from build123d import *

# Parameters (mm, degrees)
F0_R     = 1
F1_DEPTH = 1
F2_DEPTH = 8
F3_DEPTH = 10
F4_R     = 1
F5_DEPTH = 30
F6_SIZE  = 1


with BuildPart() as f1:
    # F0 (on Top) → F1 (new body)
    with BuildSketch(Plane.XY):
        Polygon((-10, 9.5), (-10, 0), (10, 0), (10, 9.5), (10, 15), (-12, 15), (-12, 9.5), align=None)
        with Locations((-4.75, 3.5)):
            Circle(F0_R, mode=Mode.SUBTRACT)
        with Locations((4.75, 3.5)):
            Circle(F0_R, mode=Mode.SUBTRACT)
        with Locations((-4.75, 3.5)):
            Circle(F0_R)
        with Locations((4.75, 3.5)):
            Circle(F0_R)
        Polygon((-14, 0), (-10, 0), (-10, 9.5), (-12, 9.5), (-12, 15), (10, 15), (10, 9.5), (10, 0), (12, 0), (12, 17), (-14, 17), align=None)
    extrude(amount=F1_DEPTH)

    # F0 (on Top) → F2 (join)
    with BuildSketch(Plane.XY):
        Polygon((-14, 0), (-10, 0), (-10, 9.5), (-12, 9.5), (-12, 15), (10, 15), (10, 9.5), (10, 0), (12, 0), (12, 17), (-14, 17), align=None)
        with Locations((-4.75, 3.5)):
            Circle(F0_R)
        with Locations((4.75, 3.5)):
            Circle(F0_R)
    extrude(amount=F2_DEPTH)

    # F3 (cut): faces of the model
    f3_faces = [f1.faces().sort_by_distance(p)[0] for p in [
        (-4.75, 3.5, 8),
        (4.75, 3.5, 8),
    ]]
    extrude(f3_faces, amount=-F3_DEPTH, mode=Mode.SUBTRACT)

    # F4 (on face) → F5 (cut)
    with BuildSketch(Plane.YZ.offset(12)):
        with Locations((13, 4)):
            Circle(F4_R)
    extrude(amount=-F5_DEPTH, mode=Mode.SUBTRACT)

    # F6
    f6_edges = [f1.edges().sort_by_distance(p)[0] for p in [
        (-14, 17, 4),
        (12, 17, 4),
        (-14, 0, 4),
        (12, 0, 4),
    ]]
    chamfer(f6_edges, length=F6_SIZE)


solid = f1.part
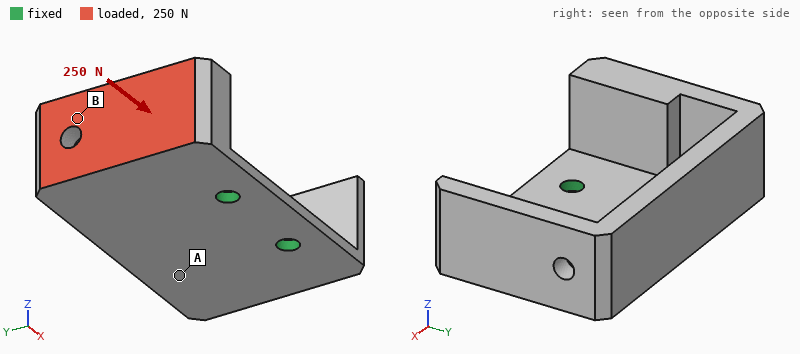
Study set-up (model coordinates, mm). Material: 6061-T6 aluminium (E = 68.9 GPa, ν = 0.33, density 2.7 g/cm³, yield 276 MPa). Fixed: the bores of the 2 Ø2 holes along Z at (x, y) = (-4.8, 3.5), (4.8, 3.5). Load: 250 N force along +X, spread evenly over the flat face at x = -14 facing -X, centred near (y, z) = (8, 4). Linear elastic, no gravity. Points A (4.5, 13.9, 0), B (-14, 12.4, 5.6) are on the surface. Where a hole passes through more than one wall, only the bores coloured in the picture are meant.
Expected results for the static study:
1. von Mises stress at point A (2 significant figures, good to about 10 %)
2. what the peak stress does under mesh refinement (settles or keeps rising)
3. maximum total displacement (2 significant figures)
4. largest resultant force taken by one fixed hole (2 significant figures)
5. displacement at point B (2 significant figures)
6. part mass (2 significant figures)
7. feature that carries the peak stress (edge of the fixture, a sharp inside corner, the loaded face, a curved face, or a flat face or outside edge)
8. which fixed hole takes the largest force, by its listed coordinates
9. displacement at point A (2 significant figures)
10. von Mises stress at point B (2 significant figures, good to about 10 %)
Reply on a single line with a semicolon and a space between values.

24 MPa; keeps rising; 0.20 mm; 220 N; 0.18 mm; 3.6 g; edge of the fixture; (-4.8, 3.5); 0.044 mm; 60 MPa
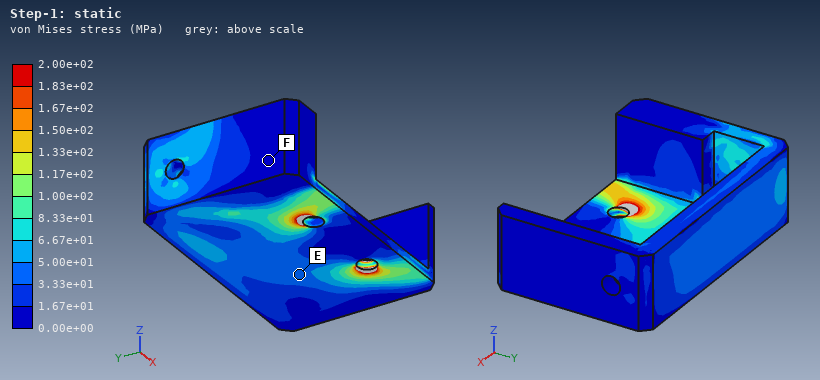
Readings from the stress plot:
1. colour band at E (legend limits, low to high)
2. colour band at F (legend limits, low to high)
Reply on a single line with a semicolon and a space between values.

3.33e+01 to 5.00e+01 MPa; 0.00e+00 to 1.67e+01 MPa
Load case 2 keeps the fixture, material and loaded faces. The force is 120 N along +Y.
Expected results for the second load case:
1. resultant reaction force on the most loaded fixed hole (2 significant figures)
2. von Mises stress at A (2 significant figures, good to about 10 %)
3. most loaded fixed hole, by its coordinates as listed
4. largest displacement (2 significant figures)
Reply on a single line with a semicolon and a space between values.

210 N; 24 MPa; (-4.8, 3.5); 0.15 mm
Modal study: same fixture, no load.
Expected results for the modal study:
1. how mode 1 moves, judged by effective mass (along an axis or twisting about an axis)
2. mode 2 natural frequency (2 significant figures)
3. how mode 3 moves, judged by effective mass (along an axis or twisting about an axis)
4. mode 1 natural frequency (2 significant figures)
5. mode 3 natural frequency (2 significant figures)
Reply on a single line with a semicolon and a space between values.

along Z; 3000 Hz; along Z; 2300 Hz; 8200 Hz
